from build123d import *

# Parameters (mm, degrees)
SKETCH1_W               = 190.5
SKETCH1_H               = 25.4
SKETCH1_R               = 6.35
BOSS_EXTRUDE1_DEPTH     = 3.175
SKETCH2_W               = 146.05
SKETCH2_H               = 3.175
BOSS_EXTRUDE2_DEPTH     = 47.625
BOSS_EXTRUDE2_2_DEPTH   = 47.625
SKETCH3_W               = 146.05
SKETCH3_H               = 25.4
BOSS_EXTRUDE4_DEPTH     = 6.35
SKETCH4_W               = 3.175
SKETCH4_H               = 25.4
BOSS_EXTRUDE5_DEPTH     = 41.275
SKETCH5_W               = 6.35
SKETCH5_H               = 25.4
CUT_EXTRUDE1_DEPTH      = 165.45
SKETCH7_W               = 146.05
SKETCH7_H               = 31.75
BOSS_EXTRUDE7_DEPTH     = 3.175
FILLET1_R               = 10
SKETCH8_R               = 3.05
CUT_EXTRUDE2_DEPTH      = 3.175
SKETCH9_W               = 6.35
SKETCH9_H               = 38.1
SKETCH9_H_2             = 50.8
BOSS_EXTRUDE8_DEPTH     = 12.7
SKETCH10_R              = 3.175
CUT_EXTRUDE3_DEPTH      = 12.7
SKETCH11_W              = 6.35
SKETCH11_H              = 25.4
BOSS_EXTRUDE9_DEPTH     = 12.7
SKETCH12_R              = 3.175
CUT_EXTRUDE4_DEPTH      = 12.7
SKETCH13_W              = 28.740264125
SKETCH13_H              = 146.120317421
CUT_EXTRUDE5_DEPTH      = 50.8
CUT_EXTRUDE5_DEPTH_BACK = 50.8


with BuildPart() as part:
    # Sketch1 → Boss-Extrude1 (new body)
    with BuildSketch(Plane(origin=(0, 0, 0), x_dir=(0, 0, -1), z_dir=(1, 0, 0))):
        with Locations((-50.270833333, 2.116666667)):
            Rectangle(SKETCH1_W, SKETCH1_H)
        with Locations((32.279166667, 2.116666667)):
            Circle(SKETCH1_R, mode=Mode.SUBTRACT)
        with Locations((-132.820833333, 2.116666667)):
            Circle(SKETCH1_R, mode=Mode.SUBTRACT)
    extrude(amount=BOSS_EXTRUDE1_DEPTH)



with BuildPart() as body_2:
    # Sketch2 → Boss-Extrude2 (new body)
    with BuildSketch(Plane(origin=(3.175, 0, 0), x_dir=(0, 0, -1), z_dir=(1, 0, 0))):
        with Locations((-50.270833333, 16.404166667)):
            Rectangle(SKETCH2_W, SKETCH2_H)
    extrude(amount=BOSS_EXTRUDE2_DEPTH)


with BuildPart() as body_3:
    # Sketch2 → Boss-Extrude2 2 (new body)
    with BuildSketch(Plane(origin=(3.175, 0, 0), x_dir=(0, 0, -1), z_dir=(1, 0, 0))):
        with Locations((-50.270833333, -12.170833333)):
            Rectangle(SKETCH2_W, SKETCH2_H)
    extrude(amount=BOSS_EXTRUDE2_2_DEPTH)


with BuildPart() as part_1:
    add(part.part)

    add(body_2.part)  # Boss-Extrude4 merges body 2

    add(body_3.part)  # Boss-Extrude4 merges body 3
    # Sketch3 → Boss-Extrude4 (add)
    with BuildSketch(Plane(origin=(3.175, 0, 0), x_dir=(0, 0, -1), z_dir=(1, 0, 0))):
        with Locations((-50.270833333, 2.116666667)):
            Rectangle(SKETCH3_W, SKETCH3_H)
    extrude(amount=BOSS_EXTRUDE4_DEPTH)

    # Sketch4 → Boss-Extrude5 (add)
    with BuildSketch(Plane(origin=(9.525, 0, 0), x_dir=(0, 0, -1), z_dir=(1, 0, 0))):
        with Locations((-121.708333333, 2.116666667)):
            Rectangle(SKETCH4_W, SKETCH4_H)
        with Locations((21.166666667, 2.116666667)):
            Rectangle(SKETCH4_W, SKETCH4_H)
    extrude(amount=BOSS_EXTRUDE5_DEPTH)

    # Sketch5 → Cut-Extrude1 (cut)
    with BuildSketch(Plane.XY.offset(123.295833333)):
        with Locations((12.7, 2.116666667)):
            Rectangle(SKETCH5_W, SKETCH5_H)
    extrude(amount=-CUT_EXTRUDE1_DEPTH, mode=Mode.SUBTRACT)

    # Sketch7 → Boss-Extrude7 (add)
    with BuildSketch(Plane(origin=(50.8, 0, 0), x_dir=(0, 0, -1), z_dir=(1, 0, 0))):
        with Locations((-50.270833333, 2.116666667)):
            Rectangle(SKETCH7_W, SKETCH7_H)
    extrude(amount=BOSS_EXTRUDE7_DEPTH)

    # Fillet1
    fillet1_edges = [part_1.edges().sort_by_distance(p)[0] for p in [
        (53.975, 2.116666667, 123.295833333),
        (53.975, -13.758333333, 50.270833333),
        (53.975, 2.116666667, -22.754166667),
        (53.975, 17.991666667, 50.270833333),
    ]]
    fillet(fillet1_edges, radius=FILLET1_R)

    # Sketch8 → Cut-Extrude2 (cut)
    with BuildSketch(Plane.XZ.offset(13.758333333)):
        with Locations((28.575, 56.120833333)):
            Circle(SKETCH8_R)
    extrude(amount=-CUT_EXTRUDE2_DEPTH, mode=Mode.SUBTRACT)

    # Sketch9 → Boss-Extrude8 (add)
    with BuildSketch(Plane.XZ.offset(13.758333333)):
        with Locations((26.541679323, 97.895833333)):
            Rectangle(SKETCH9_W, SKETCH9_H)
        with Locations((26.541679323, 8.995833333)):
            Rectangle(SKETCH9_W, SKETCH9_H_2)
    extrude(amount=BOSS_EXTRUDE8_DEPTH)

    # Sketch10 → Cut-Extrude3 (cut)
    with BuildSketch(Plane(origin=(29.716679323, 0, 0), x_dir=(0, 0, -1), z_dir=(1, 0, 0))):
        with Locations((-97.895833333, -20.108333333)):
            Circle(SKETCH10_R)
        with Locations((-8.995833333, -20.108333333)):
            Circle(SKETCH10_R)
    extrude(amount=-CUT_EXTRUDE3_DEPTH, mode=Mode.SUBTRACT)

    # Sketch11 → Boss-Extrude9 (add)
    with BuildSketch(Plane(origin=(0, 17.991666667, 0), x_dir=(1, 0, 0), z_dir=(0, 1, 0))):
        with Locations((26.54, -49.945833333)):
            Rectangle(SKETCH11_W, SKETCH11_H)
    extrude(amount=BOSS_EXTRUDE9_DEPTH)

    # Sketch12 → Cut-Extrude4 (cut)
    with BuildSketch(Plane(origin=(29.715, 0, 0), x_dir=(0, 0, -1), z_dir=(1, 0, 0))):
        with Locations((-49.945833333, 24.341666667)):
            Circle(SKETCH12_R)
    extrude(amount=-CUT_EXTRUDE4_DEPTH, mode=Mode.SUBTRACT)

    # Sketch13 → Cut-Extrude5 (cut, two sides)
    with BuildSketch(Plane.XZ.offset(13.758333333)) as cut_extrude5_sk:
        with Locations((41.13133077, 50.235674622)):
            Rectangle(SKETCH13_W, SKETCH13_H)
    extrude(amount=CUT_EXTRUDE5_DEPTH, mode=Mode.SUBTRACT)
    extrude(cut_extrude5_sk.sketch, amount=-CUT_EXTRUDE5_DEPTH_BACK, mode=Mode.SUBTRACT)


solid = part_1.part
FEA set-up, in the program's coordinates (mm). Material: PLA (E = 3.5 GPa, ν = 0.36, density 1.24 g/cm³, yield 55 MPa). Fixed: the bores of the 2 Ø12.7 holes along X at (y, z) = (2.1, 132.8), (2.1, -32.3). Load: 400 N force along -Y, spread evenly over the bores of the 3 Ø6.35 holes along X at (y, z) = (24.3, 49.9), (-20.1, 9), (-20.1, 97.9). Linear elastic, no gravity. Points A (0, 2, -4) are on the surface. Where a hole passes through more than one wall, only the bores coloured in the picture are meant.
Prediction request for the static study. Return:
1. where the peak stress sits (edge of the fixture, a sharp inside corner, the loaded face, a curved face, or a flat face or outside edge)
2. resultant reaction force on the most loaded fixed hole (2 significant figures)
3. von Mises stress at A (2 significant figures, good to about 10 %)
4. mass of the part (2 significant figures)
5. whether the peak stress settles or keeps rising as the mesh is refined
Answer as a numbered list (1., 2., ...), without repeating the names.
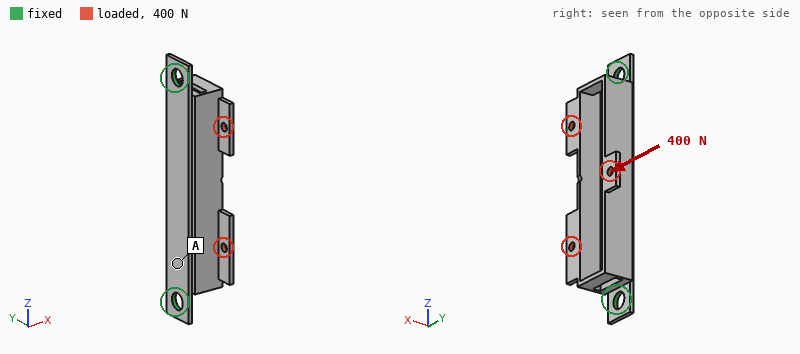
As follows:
1. edge of the fixture
2. 210 N
3. 5.1 MPa
4. 82 g
5. keeps rising
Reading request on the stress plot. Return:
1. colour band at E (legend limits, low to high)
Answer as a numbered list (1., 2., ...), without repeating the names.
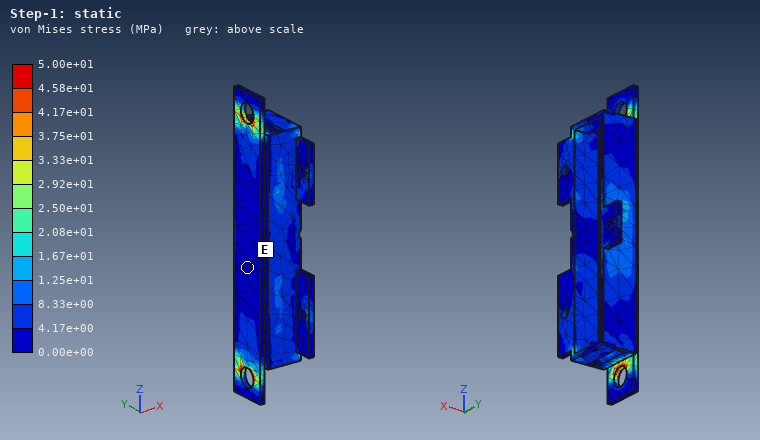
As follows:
1. 0.00e+00 to 4.17e+00 MPa
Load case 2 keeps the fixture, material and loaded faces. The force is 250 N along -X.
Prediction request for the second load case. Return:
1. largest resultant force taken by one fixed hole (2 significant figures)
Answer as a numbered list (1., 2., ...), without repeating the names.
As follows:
1. 270 N
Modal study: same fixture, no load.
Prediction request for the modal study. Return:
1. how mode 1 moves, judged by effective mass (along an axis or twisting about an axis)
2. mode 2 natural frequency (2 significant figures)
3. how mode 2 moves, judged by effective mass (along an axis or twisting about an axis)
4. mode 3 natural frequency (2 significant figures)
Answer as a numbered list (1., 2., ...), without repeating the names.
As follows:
1. along Y
2. 820 Hz
3. along X
4. 1100 Hz
